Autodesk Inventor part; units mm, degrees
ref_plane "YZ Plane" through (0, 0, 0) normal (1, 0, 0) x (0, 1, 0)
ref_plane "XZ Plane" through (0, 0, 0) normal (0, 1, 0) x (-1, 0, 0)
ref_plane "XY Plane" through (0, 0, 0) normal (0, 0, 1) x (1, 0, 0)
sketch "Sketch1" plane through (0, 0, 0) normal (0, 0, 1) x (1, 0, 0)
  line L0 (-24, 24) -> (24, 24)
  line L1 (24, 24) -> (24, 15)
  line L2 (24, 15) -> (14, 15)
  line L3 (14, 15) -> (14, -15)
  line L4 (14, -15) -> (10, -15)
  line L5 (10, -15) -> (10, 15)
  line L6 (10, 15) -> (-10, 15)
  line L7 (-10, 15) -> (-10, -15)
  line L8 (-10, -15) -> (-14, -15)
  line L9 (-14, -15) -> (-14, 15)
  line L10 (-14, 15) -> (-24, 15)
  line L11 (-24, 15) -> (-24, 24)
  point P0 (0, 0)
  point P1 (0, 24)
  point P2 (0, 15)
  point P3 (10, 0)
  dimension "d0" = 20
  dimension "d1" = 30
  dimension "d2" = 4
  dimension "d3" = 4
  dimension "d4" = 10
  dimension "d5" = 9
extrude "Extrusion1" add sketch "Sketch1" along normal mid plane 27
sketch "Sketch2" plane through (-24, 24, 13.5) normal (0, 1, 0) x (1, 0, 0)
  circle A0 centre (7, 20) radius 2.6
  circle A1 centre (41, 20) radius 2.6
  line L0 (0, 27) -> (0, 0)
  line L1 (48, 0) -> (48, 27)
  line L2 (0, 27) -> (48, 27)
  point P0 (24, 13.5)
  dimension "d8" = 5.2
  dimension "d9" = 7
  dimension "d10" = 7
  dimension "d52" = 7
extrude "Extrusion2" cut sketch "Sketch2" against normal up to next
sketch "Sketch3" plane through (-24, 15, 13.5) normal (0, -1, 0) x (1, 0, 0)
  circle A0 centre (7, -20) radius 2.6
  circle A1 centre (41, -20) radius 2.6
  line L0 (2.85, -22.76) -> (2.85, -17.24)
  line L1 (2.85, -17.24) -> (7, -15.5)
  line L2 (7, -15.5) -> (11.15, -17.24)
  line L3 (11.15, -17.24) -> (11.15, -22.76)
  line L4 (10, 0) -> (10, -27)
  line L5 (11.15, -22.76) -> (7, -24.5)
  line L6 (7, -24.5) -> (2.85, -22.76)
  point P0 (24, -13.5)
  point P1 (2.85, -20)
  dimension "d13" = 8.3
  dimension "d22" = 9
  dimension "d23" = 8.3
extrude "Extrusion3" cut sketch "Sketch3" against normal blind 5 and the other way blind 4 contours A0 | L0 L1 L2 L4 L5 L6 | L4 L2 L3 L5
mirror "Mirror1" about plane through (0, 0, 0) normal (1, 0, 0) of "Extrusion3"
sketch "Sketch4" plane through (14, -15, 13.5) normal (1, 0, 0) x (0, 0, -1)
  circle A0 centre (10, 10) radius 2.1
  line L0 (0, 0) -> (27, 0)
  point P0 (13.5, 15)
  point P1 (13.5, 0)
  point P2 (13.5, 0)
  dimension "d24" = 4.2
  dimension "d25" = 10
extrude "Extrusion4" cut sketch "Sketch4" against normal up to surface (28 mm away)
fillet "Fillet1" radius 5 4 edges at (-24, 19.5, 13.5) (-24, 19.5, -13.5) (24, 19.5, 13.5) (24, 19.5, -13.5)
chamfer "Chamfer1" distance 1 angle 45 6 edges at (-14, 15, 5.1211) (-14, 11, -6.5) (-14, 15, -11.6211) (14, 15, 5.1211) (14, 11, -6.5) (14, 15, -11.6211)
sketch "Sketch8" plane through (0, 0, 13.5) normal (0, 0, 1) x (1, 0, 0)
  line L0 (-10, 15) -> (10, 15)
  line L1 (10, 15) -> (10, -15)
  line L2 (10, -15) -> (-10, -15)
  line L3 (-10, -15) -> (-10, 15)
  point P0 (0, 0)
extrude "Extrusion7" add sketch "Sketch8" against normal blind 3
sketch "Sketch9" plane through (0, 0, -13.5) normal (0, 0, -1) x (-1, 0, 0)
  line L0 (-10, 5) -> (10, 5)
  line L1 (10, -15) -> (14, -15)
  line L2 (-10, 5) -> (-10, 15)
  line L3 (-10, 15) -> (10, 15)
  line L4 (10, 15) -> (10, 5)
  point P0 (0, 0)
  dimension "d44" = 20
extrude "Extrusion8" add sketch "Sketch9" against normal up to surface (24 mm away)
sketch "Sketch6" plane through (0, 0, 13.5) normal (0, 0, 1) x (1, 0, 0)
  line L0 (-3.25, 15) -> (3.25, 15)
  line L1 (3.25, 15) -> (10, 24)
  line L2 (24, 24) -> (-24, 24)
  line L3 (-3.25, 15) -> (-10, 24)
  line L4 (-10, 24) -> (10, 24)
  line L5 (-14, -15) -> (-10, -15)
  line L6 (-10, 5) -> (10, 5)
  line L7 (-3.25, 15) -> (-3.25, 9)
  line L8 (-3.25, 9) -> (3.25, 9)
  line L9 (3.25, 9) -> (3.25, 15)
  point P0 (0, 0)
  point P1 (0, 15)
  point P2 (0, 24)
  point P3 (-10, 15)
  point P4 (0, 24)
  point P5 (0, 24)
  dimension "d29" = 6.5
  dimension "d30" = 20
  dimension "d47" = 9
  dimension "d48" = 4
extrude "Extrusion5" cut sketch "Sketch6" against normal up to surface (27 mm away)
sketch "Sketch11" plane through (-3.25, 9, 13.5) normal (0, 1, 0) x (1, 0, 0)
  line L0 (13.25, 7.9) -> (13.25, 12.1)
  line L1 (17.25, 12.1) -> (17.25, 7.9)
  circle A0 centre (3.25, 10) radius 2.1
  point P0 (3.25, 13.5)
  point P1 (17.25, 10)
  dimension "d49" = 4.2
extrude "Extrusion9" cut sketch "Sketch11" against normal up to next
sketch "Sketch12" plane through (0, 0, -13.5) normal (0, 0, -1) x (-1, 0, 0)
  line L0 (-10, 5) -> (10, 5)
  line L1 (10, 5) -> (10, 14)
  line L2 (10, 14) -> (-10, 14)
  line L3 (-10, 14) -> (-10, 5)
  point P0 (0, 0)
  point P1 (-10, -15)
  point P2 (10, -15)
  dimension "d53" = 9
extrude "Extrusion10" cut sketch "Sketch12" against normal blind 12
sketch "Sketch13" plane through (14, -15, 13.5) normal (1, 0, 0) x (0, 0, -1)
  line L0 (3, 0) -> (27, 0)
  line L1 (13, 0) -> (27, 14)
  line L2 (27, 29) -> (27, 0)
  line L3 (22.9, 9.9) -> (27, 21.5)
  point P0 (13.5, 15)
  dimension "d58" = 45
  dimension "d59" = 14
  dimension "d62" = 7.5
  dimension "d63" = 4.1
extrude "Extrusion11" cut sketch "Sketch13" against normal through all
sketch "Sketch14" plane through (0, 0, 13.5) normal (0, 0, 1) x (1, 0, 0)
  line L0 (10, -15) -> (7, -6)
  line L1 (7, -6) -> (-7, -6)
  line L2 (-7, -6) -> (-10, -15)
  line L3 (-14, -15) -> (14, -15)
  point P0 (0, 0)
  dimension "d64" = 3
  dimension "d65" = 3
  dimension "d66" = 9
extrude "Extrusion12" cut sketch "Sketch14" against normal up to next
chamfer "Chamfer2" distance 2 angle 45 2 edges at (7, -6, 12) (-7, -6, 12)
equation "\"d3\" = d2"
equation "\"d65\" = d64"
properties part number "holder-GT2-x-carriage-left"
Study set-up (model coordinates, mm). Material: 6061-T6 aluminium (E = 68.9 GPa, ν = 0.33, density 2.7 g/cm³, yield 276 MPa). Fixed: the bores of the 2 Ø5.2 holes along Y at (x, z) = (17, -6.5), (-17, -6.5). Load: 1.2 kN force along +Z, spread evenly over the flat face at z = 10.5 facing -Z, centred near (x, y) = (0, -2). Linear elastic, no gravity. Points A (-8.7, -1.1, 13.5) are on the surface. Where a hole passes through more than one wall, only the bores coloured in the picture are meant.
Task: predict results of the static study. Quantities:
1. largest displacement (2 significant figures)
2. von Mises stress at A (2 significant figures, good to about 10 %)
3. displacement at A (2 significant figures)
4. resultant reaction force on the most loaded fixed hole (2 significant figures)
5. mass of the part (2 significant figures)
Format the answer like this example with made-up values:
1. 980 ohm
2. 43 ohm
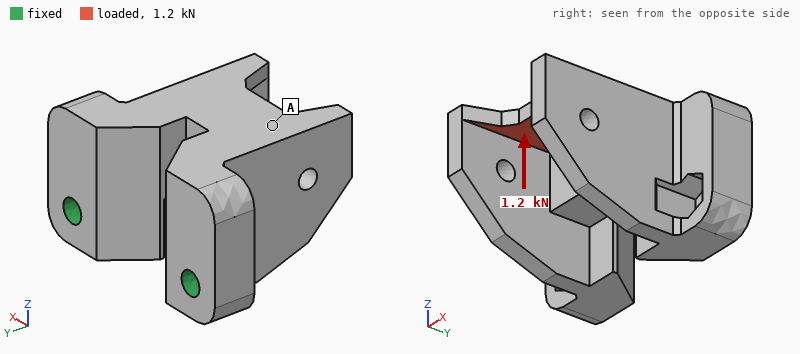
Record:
1. 0.14 mm
2. 32 MPa
3. 0.11 mm
4. 600 N
5. 44 g
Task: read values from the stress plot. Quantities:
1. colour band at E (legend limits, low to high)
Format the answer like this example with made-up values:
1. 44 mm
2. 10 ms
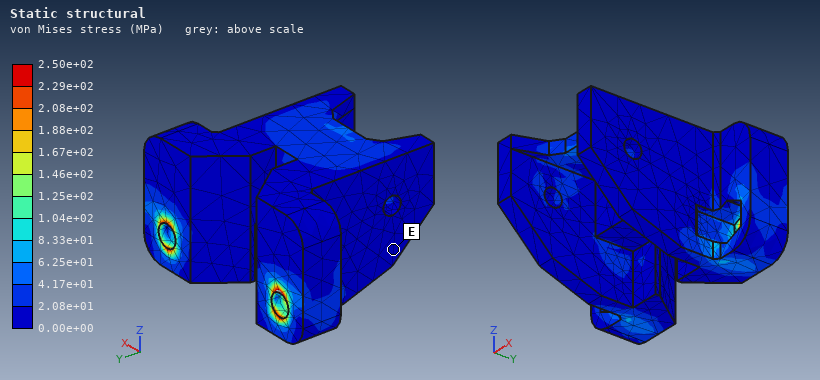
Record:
1. 0.00e+00 to 2.08e+01 MPa
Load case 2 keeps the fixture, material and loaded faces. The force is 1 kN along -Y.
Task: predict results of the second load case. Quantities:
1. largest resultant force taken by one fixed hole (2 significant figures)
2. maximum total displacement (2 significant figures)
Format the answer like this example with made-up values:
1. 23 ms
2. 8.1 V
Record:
1. 540 N
2. 80 µm
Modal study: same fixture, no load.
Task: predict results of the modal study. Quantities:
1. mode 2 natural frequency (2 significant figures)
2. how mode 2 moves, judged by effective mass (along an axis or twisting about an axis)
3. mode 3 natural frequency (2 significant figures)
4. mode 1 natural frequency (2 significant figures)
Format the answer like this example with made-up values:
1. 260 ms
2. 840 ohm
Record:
1. 6300 Hz
2. along X
3. 10 kHz
4. 3800 Hz
